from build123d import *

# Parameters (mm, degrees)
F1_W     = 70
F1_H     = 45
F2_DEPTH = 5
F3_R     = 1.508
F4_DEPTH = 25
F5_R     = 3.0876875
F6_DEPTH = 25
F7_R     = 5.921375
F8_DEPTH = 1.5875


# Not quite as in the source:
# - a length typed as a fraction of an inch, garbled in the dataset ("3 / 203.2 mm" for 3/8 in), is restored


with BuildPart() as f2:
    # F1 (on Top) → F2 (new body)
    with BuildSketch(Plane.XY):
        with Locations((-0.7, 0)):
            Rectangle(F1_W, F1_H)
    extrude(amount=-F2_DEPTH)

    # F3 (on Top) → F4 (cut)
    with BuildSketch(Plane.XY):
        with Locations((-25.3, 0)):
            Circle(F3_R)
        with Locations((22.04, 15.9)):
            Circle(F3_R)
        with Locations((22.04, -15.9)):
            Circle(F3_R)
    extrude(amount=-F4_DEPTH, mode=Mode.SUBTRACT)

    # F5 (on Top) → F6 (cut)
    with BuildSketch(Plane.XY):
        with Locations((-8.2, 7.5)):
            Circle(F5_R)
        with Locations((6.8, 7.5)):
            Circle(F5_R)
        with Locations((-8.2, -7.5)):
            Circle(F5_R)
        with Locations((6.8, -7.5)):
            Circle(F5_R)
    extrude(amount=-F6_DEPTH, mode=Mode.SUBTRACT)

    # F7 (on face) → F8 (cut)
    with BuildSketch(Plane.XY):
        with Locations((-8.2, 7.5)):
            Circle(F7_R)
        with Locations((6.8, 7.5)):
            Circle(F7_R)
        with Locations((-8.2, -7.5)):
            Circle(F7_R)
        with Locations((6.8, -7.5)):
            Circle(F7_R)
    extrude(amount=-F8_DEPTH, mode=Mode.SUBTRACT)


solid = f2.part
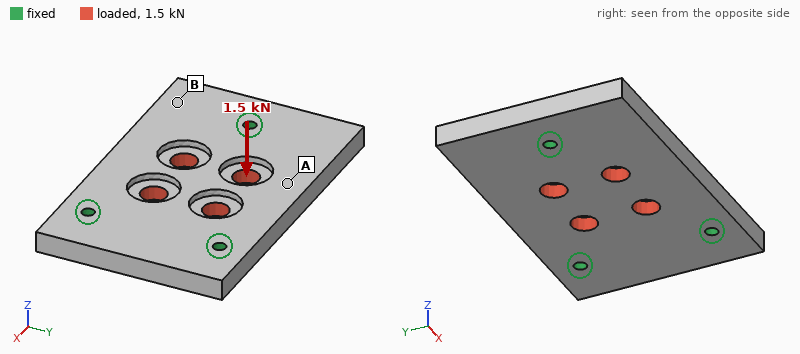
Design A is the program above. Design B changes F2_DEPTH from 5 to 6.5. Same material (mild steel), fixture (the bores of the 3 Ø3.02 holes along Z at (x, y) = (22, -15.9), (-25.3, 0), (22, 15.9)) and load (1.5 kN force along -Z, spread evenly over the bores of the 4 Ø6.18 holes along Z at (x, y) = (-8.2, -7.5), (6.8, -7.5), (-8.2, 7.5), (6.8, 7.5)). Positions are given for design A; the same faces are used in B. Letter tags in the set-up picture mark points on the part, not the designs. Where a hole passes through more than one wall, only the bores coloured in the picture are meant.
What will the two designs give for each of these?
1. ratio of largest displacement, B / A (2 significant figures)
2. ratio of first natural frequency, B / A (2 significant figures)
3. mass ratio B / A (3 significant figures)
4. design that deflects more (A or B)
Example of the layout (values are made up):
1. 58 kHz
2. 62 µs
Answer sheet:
1. 0.50
2. 1.2
3. 1.31
4. A
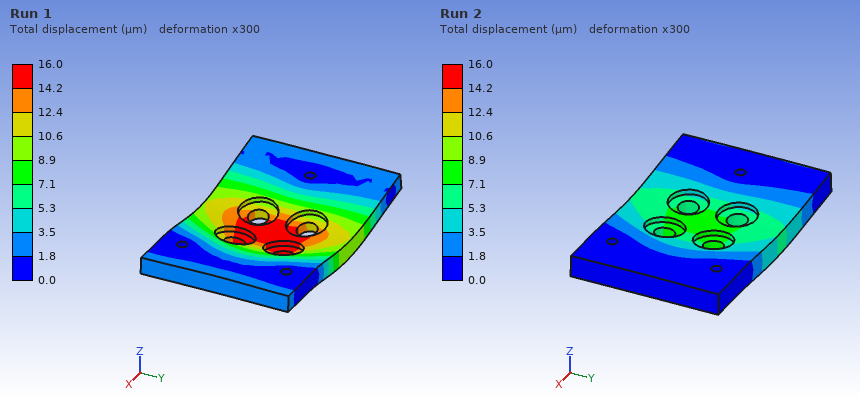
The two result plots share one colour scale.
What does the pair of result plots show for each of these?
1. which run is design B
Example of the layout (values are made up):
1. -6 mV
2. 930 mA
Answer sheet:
1. Run 2
